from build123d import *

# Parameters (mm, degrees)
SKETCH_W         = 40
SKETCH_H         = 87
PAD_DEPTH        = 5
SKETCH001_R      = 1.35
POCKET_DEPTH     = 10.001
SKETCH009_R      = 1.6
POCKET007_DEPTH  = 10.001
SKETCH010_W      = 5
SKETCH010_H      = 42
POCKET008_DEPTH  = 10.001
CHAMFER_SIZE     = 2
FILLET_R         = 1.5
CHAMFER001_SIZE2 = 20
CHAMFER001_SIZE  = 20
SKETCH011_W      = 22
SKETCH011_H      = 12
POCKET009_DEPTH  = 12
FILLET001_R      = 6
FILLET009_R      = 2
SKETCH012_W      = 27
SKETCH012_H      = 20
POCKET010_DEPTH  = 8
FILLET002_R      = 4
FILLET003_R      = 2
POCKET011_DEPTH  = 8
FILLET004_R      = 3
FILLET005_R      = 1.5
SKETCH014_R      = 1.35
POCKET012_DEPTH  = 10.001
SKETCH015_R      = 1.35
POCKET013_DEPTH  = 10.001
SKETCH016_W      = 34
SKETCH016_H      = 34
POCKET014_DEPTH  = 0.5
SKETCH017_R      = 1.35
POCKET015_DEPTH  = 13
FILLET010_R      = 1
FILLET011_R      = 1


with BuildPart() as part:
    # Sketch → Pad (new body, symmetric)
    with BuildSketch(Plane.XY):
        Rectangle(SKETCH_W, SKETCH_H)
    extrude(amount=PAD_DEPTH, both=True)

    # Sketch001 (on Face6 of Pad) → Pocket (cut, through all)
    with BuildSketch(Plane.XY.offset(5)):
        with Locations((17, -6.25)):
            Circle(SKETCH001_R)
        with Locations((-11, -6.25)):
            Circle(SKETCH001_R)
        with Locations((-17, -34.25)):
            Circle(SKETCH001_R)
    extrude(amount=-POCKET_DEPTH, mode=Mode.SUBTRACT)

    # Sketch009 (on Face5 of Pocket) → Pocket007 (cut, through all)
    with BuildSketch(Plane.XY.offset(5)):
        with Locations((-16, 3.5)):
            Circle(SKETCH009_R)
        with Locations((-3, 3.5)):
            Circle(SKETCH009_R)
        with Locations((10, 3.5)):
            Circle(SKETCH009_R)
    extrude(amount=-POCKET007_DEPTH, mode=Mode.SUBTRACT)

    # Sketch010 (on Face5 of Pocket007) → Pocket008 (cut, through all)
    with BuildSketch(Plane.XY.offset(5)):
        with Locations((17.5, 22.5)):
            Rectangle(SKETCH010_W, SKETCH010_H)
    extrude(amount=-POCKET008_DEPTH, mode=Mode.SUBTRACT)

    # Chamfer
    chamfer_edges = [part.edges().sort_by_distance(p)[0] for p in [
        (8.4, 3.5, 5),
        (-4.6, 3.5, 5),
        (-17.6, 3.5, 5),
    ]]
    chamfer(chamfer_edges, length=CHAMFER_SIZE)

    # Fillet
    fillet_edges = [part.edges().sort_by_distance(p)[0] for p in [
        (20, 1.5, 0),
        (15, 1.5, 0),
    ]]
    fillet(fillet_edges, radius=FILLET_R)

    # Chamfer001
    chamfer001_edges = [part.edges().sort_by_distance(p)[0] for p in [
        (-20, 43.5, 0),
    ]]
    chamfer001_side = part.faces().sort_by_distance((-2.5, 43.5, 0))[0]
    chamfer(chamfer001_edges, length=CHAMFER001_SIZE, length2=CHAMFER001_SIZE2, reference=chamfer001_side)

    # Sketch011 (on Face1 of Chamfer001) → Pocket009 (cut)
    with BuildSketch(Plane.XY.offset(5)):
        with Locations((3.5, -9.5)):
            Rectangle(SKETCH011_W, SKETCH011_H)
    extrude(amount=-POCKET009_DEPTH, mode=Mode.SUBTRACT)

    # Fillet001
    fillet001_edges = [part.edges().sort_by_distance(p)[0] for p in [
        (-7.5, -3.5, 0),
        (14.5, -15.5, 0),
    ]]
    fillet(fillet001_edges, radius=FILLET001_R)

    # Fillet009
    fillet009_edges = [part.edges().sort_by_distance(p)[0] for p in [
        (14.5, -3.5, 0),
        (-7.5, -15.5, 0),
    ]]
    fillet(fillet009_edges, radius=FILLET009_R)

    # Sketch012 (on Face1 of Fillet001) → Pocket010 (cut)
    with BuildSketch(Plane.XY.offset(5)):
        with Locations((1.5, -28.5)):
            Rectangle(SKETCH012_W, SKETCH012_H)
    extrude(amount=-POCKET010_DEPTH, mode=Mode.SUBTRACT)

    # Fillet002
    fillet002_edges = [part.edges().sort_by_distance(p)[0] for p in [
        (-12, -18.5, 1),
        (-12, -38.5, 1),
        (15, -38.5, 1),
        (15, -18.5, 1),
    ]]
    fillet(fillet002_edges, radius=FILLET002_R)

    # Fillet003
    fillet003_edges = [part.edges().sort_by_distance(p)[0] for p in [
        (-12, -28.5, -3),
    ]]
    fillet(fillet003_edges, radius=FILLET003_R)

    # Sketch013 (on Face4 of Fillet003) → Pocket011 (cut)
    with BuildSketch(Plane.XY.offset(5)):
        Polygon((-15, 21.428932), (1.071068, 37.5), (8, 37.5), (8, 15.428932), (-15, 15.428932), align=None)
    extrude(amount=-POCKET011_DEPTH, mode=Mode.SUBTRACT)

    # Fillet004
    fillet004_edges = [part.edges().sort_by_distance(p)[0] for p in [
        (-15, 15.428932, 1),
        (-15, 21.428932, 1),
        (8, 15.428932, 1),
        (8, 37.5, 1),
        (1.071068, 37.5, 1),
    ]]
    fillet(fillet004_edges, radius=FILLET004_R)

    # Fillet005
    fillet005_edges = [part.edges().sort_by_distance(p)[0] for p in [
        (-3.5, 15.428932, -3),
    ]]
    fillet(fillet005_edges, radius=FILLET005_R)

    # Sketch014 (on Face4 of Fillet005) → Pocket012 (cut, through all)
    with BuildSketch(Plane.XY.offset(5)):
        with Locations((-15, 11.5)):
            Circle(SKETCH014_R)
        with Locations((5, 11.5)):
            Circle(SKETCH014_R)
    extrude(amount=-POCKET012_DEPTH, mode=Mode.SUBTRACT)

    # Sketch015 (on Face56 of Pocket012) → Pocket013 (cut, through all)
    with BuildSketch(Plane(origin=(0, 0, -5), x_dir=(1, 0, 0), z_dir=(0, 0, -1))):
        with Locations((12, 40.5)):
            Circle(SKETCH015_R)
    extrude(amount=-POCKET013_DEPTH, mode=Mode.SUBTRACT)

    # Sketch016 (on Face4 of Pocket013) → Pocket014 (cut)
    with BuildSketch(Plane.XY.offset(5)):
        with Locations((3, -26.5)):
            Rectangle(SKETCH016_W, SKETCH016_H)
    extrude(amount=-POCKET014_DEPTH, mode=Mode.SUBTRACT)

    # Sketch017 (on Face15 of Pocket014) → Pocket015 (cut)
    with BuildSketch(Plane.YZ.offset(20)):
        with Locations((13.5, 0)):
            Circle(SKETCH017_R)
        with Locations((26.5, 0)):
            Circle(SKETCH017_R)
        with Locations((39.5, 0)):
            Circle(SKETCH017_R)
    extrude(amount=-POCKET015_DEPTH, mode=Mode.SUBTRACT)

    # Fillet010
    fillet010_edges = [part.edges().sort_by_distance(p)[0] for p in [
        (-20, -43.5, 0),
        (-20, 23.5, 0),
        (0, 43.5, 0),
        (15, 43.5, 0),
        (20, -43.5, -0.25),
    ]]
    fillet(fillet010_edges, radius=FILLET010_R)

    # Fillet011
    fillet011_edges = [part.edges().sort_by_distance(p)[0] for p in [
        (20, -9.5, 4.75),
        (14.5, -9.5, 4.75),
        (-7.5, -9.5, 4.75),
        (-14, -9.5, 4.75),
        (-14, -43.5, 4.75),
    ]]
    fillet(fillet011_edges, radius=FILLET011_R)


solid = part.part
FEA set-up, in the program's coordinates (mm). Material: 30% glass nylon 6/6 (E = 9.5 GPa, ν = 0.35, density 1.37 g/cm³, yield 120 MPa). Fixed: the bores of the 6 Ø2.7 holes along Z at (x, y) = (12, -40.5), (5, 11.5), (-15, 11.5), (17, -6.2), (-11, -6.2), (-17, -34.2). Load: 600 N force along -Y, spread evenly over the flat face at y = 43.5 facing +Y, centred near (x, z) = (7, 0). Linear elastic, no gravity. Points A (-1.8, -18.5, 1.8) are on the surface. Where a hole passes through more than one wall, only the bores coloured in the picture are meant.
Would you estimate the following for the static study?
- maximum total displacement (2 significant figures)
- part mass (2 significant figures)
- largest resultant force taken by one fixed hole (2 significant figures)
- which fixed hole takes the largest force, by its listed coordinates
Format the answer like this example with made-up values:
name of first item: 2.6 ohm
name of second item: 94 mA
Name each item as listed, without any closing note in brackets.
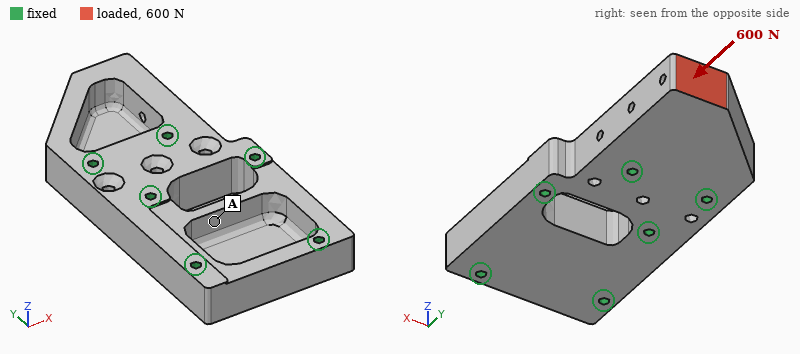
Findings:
maximum total displacement: 62 µm
part mass: 28 g
largest resultant force taken by one fixed hole: 430 N
which fixed hole takes the largest force, by its listed coordinates: (5, 11.5)
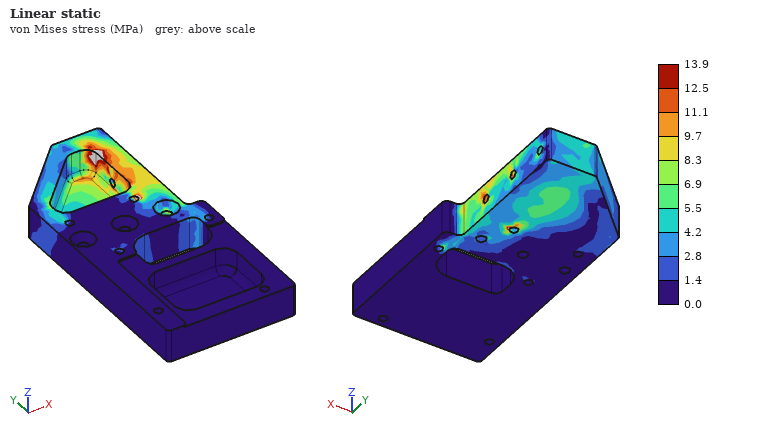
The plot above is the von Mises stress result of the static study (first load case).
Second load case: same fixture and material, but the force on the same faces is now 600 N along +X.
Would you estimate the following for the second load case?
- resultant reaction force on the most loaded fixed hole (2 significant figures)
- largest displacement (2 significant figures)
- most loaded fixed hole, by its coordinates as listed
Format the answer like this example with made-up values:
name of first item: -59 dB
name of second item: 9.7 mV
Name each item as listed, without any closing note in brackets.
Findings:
resultant reaction force on the most loaded fixed hole: 730 N
largest displacement: 0.14 mm
most loaded fixed hole, by its coordinates as listed: (-15, 11.5)
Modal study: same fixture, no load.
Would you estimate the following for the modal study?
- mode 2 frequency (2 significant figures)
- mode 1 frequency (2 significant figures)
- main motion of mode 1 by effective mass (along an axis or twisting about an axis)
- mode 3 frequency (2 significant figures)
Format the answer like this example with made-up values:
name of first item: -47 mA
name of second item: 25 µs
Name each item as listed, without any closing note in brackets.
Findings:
mode 2 frequency: 6600 Hz
mode 1 frequency: 3300 Hz
main motion of mode 1 by effective mass: along Z
mode 3 frequency: 9000 Hz
